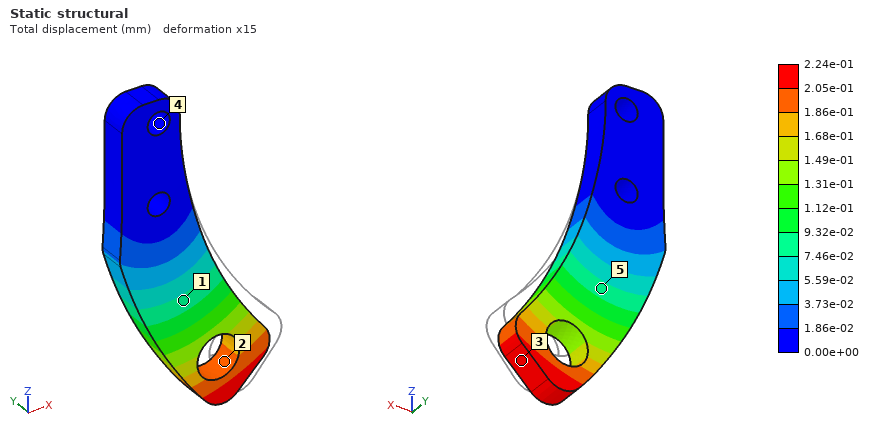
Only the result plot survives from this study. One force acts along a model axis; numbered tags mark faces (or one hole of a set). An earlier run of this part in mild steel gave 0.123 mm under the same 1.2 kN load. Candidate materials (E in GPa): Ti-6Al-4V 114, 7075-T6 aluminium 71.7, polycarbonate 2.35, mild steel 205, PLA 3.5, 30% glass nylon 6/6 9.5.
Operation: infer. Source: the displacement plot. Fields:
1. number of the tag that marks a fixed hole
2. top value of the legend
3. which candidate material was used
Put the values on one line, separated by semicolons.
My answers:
4; 2.24e-01 mm; Ti-6Al-4V
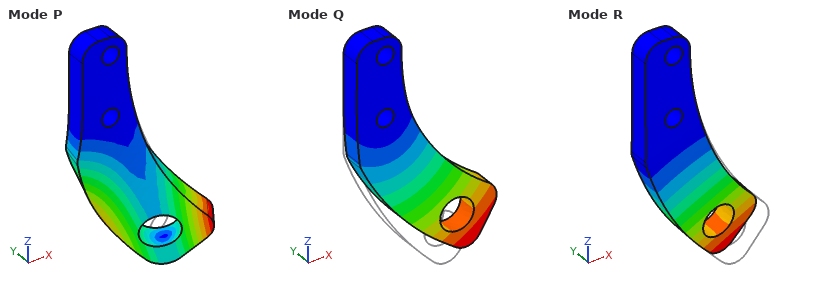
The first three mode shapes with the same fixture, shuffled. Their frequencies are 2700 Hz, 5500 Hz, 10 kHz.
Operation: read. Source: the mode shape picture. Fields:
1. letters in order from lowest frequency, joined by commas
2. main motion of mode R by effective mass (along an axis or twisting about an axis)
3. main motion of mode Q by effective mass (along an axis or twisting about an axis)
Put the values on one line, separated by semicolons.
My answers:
R, Q, P; along Y; along X
